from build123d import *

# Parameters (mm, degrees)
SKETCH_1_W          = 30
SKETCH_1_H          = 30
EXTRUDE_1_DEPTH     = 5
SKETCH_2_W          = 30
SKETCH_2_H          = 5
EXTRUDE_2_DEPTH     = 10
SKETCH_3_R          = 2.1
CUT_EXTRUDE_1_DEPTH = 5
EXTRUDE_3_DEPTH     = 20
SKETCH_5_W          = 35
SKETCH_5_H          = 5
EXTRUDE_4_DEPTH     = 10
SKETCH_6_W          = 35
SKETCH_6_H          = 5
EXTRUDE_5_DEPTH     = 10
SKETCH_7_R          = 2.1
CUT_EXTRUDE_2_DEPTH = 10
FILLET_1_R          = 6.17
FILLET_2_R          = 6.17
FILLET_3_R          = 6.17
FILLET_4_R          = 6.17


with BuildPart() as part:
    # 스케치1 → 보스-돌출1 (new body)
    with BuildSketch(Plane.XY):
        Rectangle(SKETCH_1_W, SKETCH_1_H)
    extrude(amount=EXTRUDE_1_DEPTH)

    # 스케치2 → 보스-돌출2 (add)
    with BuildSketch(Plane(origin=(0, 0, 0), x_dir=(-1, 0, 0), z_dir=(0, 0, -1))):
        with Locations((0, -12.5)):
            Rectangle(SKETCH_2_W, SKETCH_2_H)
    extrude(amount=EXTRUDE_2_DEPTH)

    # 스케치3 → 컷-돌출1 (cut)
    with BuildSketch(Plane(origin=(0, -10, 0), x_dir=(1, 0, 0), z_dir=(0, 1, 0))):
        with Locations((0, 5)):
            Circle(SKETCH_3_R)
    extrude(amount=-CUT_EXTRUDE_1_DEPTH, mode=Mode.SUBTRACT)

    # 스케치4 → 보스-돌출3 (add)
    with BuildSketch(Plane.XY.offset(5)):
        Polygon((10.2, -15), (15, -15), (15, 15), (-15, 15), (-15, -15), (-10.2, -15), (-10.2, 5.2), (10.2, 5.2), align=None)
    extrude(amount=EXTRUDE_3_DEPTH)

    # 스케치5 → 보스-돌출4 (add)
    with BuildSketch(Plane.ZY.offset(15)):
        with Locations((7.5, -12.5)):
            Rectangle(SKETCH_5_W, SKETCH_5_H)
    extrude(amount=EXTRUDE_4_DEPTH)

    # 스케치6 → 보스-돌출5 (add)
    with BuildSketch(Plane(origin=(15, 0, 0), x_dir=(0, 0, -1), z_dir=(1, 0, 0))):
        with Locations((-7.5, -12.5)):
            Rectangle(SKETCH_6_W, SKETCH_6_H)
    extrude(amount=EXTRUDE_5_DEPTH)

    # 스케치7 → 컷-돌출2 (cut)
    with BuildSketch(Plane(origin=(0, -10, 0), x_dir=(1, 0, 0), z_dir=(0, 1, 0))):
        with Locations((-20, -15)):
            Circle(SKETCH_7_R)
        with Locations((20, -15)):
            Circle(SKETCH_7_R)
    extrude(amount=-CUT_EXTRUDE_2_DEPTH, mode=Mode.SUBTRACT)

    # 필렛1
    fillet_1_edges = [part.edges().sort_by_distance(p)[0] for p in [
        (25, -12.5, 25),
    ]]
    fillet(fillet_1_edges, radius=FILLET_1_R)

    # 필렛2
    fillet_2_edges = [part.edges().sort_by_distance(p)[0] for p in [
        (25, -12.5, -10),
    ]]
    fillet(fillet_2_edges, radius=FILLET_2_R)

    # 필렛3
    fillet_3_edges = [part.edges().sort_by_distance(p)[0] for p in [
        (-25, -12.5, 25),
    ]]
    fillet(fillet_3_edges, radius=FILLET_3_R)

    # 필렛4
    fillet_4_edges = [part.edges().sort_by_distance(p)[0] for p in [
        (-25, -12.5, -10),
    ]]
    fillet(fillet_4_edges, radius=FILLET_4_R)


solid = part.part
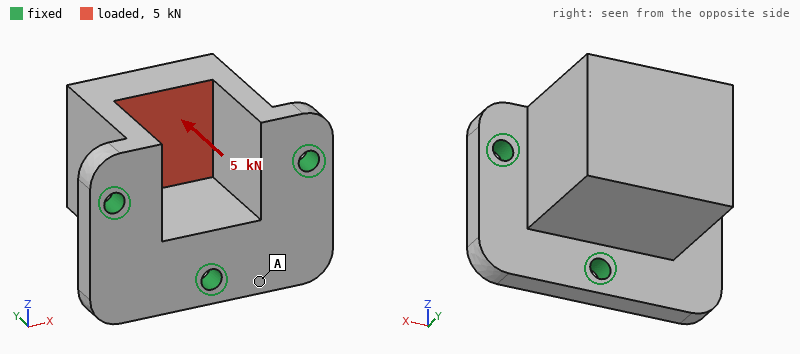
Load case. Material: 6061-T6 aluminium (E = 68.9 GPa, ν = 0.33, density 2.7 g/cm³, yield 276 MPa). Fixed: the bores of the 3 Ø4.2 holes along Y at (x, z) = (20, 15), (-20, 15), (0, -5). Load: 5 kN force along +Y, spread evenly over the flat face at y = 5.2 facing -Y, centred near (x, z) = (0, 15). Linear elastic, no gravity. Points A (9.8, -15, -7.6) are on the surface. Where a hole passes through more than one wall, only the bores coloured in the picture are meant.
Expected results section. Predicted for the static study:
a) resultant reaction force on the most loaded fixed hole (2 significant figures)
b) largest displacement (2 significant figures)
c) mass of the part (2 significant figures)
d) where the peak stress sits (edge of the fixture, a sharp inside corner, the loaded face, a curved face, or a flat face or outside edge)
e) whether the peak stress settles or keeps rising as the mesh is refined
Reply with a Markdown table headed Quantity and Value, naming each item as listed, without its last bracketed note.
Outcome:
| Quantity | Value |
|---|---|
| resultant reaction force on the most loaded fixed hole | 2.4 kN |
| largest displacement | 57 µm |
| mass of the part | 51 g |
| where the peak stress sits | edge of the fixture |
| whether the peak stress settles or keeps rising as the mesh is refined | keeps rising |
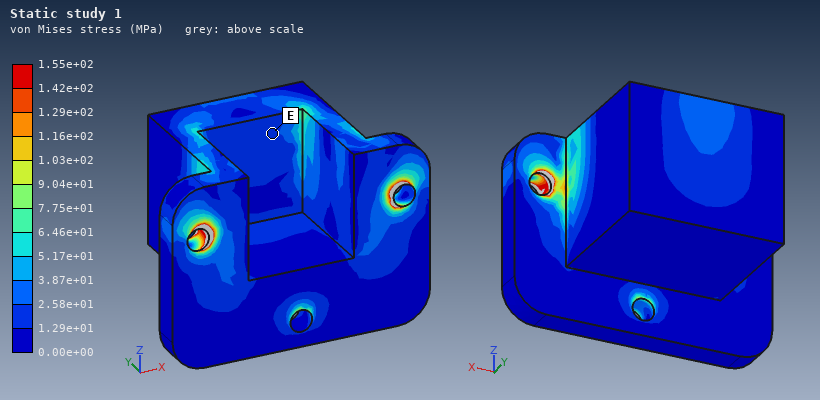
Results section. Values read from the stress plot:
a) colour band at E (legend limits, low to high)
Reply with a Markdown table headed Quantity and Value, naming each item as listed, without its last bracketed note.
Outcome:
| Quantity | Value |
|---|---|
| colour band at E | 1.29e+01 to 2.58e+01 MPa |
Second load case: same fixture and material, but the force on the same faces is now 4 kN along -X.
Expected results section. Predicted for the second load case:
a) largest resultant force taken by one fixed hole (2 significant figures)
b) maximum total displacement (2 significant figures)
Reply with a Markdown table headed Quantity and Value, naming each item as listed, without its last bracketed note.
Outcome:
| Quantity | Value |
|---|---|
| largest resultant force taken by one fixed hole | 2.1 kN |
| maximum total displacement | 0.11 mm |
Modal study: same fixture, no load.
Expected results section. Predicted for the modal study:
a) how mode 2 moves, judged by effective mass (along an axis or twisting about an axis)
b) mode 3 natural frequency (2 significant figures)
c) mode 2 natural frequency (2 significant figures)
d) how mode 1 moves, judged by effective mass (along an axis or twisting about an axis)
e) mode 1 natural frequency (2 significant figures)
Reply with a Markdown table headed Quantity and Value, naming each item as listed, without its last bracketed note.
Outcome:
| Quantity | Value |
|---|---|
| how mode 2 moves, judged by effective mass | along X |
| mode 3 natural frequency | 13 kHz |
| mode 2 natural frequency | 7300 Hz |
| how mode 1 moves, judged by effective mass | along Z |
| mode 1 natural frequency | 6600 Hz |
